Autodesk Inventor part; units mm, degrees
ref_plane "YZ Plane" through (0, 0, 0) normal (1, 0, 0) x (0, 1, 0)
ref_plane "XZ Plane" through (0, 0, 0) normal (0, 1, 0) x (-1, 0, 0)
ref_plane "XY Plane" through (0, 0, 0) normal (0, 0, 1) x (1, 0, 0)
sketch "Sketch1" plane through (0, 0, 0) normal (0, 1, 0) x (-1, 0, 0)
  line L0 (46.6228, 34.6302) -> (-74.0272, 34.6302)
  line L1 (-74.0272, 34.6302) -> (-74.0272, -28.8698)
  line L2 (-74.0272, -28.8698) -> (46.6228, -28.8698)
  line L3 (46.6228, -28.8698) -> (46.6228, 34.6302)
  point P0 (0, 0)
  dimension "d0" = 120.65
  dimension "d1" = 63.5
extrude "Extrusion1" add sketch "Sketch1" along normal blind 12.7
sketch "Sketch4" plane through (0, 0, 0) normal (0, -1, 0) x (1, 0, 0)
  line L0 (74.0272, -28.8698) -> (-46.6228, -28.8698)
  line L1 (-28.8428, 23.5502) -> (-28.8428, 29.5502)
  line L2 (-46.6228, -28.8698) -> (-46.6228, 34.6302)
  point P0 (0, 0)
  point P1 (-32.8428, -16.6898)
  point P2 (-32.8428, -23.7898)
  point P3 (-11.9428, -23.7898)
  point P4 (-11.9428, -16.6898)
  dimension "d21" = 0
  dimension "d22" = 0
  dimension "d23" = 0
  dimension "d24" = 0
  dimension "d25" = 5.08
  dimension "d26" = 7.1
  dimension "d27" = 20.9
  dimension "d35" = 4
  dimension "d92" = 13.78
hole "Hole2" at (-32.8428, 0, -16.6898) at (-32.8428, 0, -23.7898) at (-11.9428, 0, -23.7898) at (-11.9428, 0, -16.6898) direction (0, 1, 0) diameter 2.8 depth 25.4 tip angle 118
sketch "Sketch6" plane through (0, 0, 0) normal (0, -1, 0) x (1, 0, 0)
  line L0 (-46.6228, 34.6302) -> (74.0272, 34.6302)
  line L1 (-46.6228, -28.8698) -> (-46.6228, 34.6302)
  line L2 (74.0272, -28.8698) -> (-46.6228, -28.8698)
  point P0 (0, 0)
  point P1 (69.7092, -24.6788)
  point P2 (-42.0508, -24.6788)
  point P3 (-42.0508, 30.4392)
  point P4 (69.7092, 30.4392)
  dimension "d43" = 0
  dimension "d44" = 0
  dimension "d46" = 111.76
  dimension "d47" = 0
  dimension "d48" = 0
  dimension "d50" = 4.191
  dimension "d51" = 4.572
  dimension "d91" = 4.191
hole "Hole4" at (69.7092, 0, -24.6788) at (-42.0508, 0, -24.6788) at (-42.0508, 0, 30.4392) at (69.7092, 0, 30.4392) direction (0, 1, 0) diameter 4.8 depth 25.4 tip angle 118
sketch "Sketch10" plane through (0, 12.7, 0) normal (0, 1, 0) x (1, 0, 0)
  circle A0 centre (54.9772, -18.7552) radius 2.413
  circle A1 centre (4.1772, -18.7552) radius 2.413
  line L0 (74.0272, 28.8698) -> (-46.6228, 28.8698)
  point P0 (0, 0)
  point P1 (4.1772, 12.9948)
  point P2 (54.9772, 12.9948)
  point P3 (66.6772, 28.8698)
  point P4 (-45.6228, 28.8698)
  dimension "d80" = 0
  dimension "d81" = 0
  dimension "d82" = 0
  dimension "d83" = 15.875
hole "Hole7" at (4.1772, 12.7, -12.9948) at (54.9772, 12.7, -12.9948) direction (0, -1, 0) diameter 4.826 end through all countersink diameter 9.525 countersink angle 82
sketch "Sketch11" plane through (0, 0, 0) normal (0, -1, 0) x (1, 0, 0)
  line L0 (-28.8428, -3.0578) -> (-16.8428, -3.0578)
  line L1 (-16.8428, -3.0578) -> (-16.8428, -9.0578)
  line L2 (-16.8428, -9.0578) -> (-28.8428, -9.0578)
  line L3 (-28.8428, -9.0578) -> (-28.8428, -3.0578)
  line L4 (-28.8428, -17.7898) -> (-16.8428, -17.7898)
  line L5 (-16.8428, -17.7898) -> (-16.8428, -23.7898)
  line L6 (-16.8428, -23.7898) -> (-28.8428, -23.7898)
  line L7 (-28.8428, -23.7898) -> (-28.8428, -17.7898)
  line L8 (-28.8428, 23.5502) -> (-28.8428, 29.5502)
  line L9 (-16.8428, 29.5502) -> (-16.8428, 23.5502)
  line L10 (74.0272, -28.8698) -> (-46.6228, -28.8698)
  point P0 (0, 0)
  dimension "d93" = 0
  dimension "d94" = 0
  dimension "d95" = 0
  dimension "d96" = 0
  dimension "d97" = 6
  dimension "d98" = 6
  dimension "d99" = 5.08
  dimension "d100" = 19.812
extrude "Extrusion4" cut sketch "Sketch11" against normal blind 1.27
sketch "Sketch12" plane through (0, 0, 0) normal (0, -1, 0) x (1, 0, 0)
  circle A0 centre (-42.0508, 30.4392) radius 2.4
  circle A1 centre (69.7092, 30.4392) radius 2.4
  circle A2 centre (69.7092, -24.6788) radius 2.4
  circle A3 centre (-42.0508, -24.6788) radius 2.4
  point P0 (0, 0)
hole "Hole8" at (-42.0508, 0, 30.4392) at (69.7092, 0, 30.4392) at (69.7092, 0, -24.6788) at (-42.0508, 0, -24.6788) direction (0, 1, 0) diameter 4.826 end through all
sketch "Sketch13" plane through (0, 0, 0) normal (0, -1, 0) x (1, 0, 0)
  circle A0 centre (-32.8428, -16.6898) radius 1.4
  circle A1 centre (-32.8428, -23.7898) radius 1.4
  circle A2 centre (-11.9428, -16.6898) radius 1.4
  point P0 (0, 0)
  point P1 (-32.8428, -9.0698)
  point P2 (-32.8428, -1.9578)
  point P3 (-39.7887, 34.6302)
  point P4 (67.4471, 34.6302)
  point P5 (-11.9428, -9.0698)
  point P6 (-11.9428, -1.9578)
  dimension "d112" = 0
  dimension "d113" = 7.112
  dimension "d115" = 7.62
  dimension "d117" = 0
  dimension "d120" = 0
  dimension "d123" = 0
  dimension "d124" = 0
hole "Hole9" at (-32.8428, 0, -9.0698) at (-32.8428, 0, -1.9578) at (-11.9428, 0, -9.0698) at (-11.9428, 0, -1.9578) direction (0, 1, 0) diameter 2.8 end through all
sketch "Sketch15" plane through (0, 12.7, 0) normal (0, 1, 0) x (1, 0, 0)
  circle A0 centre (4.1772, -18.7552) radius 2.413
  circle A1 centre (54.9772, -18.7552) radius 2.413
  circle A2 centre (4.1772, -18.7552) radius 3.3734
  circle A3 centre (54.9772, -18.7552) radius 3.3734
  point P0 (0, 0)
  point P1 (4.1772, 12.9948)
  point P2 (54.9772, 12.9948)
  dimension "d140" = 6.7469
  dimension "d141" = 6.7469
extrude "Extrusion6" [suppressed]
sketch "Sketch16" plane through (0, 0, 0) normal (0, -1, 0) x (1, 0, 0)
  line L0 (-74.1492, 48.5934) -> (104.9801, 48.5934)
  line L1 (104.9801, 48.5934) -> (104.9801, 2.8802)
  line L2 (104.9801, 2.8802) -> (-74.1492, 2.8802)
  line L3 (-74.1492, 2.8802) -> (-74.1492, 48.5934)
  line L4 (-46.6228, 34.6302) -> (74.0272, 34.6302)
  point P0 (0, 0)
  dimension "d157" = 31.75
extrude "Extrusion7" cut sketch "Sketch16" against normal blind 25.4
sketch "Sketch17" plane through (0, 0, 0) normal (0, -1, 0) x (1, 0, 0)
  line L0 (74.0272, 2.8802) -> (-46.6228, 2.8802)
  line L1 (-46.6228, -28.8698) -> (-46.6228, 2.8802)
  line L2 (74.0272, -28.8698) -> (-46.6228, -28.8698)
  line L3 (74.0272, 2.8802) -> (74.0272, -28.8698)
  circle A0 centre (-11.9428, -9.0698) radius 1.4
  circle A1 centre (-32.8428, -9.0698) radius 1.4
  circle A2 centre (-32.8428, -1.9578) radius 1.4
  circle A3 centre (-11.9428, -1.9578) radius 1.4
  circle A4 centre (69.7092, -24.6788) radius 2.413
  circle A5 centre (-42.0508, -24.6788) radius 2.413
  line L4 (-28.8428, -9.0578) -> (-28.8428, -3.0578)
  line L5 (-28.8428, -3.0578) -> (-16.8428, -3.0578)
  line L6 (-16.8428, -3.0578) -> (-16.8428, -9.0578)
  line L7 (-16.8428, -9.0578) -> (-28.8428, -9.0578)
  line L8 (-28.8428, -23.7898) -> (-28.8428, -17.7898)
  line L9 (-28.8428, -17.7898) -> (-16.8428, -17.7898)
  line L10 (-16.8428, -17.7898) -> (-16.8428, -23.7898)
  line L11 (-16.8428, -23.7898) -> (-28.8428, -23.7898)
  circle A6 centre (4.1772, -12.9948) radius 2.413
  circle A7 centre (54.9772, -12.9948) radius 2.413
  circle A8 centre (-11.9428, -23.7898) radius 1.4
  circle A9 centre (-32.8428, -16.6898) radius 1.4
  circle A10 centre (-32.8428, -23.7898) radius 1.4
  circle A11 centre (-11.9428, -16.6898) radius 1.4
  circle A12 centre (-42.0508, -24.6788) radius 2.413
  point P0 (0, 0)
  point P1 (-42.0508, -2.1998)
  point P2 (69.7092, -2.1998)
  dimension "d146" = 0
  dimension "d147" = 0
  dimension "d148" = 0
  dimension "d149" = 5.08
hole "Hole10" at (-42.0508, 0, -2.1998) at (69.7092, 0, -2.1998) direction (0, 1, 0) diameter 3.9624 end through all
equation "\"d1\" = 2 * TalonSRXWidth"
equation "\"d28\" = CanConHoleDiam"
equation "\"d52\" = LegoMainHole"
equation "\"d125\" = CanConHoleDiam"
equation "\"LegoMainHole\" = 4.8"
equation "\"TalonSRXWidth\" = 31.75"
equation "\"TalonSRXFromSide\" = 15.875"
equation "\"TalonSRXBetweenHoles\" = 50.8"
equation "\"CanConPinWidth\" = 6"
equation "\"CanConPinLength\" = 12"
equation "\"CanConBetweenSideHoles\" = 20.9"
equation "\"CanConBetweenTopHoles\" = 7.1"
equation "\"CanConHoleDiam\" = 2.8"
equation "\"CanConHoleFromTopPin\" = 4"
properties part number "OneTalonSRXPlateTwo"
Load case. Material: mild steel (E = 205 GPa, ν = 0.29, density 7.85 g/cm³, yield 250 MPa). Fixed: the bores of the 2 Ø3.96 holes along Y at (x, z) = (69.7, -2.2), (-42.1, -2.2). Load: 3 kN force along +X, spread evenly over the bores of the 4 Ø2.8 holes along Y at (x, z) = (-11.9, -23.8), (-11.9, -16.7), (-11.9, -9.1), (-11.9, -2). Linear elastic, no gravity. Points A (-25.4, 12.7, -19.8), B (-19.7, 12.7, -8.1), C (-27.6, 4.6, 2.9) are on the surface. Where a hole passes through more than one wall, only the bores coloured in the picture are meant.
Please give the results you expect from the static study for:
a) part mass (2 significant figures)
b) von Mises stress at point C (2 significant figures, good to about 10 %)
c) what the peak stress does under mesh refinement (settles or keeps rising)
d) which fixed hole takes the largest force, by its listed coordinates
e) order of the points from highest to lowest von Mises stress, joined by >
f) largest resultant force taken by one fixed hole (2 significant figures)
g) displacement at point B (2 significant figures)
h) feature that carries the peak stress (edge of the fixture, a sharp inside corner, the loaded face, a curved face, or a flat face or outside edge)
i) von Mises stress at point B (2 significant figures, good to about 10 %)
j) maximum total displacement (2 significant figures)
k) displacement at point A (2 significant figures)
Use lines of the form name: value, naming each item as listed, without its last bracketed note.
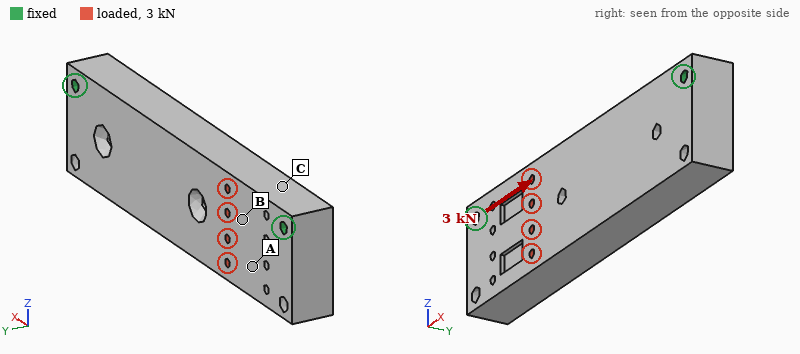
part mass: 360 g
von Mises stress at point C: 12 MPa
what the peak stress does under mesh refinement: keeps rising
which fixed hole takes the largest force, by its listed coordinates: (-42.1, -2.2)
order of the points from highest to lowest von Mises stress, joined by >: C > B > A
largest resultant force taken by one fixed hole: 1.8 kN
displacement at point B: 1.5 µm
feature that carries the peak stress: edge of the fixture
von Mises stress at point B: 6.4 MPa
maximum total displacement: 2.0 µm
displacement at point A: 1.8 µm
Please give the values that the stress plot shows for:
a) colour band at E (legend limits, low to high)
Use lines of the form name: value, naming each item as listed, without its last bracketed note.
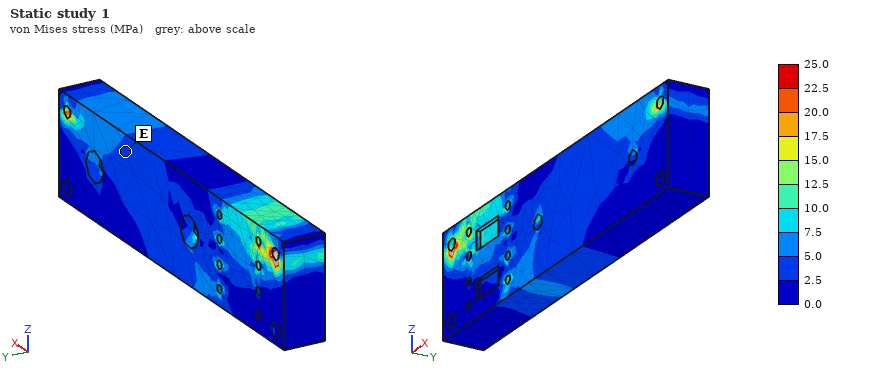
colour band at E: 2.5 to 5.0 MPa
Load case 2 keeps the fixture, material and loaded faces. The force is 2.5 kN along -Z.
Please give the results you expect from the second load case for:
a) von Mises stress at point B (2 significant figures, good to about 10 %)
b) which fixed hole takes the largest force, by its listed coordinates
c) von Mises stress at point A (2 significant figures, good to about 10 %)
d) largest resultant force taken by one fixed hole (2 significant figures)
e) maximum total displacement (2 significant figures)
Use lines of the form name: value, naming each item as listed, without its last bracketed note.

von Mises stress at point B: 10 MPa
which fixed hole takes the largest force, by its listed coordinates: (-42.1, -2.2)
von Mises stress at point A: 10 MPa
largest resultant force taken by one fixed hole: 2.2 kN
maximum total displacement: 6.3 µm
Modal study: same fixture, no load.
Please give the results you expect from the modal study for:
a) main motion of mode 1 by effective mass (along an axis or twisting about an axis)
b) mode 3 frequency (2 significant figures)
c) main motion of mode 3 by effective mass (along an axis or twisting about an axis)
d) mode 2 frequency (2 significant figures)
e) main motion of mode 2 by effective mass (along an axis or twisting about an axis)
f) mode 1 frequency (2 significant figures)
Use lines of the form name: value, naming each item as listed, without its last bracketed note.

main motion of mode 1 by effective mass: along Y
mode 3 frequency: 7100 Hz
main motion of mode 3 by effective mass: twisting about X
mode 2 frequency: 6700 Hz
main motion of mode 2 by effective mass: along Z
mode 1 frequency: 3600 Hz
